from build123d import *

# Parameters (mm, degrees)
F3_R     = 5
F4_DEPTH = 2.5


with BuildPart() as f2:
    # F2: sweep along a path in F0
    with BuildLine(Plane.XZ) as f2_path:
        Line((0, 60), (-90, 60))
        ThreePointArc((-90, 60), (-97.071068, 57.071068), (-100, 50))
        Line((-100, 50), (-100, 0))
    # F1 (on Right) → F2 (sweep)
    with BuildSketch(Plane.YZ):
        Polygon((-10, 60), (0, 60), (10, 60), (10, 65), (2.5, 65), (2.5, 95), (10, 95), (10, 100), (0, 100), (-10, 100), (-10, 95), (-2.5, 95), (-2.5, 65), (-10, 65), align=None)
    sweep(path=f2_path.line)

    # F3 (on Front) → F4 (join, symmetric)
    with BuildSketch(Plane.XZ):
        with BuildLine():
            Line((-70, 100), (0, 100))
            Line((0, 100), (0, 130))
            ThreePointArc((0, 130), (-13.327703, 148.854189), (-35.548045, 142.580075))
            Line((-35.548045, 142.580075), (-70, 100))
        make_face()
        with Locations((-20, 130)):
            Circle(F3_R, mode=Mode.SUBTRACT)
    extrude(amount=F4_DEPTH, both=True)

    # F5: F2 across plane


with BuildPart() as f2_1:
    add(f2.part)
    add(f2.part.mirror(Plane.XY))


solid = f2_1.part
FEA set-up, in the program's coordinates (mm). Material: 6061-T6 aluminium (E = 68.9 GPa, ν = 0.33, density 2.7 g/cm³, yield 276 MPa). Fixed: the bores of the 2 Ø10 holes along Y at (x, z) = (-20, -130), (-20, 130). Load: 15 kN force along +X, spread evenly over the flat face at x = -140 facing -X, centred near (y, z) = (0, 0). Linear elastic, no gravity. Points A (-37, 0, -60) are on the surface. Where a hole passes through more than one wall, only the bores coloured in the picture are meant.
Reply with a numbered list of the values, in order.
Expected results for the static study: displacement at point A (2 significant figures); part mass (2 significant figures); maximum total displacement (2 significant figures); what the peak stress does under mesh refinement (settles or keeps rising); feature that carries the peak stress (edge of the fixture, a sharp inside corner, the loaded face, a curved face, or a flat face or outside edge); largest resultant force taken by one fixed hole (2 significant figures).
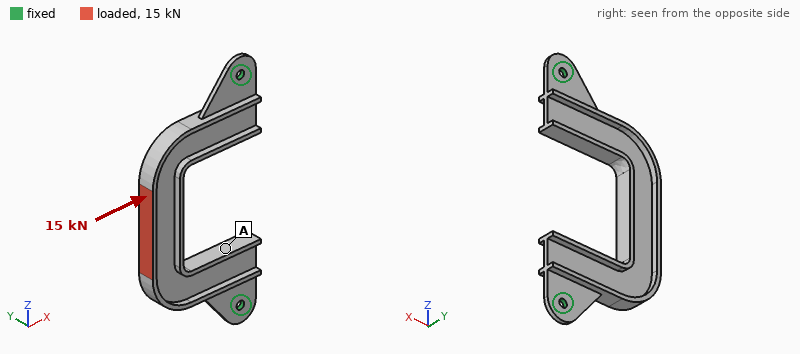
1. 0.090 mm
2. 420 g
3. 0.22 mm
4. keeps rising
5. edge of the fixture
6. 9.4 kN
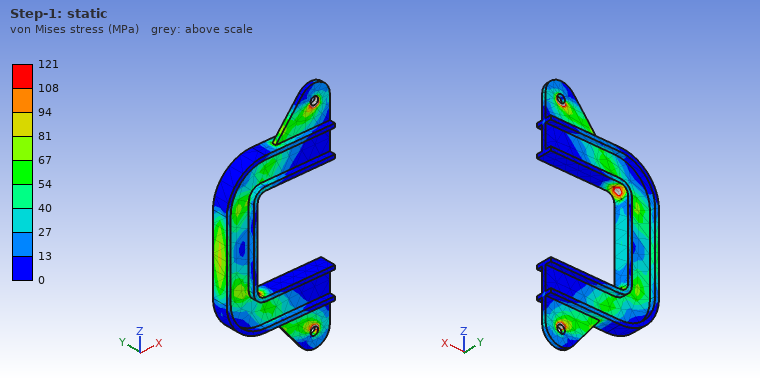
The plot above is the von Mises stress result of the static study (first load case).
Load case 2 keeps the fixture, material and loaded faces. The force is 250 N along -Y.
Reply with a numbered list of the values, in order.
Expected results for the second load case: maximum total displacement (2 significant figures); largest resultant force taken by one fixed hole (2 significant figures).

1. 1.1 mm
2. 130 N
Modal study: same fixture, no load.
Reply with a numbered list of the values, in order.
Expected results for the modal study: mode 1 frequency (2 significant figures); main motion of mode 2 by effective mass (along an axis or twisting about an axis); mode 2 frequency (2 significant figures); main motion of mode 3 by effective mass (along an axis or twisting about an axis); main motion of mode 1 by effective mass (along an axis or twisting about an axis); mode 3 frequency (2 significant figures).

1. 210 Hz
2. twisting about X
3. 580 Hz
4. along Y
5. along Y
6. 830 Hz
